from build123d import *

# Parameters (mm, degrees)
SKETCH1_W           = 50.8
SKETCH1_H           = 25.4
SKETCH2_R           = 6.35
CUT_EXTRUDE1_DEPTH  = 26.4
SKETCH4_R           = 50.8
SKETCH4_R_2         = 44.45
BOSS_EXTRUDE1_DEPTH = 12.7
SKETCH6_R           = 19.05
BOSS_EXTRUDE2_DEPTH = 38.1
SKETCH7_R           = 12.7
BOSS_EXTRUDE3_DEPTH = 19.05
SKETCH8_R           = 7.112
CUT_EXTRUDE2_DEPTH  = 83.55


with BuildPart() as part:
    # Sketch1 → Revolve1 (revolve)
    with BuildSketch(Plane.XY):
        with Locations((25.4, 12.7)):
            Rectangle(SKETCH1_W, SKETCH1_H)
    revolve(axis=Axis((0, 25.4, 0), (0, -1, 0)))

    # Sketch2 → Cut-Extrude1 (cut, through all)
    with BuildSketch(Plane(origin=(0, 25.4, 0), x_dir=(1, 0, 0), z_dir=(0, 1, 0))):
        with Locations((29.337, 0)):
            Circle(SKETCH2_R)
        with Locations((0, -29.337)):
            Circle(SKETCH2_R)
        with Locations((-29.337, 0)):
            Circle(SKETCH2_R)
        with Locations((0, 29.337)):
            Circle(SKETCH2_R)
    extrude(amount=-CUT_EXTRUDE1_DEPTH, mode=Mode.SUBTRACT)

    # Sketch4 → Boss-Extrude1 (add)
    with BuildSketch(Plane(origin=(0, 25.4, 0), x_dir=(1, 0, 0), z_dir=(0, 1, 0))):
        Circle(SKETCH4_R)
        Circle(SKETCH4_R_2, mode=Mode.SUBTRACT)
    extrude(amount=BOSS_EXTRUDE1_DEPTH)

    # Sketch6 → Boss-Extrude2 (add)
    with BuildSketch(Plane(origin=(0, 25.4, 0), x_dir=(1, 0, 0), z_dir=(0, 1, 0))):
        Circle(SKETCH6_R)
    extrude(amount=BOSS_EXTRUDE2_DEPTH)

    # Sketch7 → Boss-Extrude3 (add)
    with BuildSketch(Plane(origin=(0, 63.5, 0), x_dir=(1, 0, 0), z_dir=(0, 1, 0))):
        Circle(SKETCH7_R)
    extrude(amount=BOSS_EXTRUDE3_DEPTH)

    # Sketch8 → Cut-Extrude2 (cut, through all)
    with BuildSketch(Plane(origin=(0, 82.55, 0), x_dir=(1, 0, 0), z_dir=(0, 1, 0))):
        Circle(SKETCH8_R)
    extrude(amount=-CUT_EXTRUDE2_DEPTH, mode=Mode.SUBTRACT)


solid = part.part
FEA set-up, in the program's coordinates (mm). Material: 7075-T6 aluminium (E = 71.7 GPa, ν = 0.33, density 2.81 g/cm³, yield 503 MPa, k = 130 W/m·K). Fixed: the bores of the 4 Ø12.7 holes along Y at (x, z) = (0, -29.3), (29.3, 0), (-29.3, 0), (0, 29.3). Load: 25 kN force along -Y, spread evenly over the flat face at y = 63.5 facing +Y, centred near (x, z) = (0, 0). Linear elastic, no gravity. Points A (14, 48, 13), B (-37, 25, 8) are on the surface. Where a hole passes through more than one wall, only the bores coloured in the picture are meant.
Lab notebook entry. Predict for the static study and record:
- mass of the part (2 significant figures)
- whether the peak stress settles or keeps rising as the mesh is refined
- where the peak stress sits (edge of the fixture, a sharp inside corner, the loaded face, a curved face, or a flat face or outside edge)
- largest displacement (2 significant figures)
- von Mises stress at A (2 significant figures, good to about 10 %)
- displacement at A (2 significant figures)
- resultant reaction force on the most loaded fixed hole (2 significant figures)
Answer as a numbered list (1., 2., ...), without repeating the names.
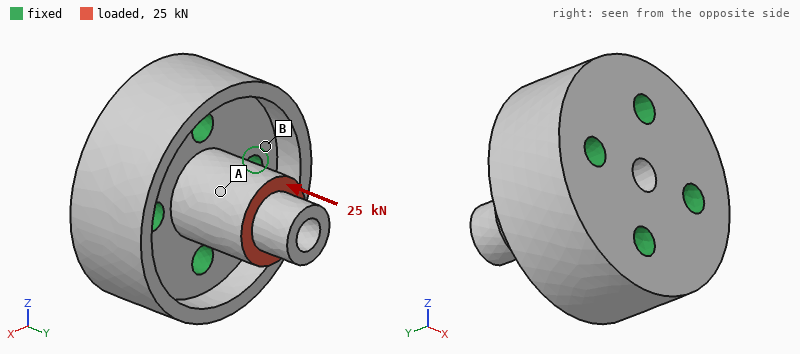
1. 720 g
2. keeps rising
3. edge of the fixture
4. 21 µm
5. 26 MPa
6. 13 µm
7. 6.7 kN
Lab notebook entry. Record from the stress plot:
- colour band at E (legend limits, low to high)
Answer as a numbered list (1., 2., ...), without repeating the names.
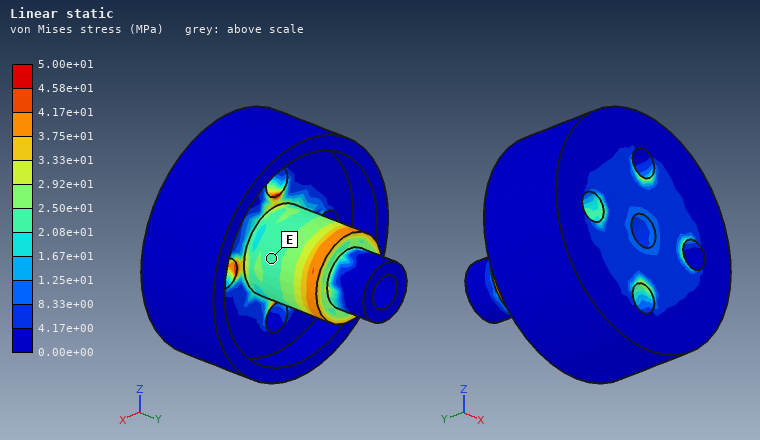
1. 2.08e+01 to 2.50e+01 MPa
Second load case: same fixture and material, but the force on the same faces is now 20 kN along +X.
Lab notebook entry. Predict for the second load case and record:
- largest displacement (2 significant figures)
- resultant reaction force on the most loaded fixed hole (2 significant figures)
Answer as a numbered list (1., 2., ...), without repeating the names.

1. 0.18 mm
2. 19 kN
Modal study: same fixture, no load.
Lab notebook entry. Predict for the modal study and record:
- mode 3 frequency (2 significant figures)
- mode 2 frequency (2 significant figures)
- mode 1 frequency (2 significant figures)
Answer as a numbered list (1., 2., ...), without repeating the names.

1. 15 kHz
2. 7700 Hz
3. 7700 Hz
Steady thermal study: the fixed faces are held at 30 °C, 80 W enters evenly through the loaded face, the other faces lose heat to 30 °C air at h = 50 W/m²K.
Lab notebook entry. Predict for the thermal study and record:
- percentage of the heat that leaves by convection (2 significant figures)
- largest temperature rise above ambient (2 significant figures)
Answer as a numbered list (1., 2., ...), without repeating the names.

1. 11 %
2. 28 K
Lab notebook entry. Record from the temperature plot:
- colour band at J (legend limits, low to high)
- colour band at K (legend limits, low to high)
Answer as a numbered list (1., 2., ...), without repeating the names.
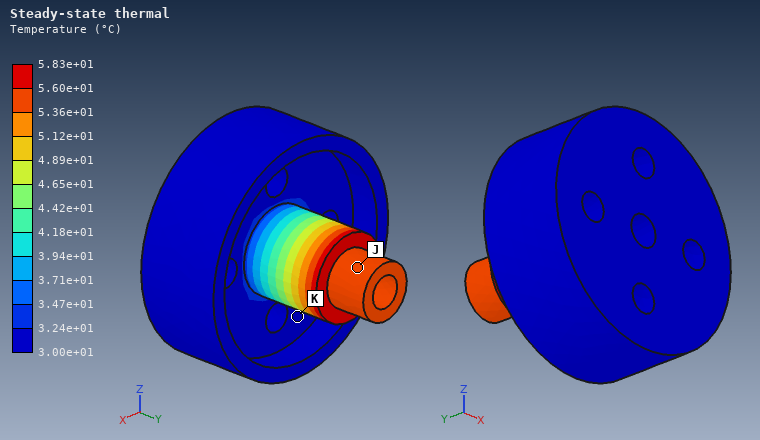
1. 5.36e+01 to 5.60e+01 °C
2. 3.00e+01 to 3.24e+01 °C
